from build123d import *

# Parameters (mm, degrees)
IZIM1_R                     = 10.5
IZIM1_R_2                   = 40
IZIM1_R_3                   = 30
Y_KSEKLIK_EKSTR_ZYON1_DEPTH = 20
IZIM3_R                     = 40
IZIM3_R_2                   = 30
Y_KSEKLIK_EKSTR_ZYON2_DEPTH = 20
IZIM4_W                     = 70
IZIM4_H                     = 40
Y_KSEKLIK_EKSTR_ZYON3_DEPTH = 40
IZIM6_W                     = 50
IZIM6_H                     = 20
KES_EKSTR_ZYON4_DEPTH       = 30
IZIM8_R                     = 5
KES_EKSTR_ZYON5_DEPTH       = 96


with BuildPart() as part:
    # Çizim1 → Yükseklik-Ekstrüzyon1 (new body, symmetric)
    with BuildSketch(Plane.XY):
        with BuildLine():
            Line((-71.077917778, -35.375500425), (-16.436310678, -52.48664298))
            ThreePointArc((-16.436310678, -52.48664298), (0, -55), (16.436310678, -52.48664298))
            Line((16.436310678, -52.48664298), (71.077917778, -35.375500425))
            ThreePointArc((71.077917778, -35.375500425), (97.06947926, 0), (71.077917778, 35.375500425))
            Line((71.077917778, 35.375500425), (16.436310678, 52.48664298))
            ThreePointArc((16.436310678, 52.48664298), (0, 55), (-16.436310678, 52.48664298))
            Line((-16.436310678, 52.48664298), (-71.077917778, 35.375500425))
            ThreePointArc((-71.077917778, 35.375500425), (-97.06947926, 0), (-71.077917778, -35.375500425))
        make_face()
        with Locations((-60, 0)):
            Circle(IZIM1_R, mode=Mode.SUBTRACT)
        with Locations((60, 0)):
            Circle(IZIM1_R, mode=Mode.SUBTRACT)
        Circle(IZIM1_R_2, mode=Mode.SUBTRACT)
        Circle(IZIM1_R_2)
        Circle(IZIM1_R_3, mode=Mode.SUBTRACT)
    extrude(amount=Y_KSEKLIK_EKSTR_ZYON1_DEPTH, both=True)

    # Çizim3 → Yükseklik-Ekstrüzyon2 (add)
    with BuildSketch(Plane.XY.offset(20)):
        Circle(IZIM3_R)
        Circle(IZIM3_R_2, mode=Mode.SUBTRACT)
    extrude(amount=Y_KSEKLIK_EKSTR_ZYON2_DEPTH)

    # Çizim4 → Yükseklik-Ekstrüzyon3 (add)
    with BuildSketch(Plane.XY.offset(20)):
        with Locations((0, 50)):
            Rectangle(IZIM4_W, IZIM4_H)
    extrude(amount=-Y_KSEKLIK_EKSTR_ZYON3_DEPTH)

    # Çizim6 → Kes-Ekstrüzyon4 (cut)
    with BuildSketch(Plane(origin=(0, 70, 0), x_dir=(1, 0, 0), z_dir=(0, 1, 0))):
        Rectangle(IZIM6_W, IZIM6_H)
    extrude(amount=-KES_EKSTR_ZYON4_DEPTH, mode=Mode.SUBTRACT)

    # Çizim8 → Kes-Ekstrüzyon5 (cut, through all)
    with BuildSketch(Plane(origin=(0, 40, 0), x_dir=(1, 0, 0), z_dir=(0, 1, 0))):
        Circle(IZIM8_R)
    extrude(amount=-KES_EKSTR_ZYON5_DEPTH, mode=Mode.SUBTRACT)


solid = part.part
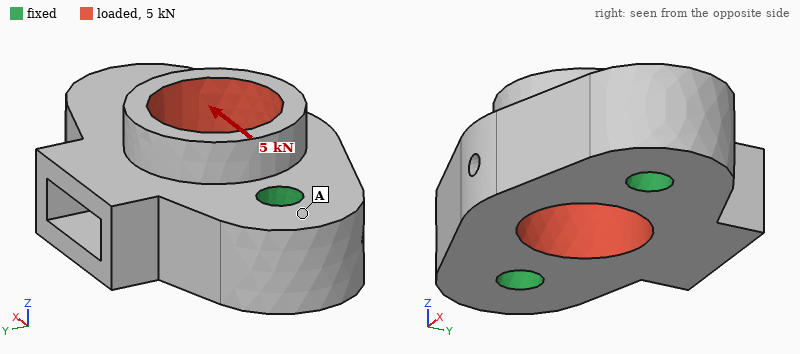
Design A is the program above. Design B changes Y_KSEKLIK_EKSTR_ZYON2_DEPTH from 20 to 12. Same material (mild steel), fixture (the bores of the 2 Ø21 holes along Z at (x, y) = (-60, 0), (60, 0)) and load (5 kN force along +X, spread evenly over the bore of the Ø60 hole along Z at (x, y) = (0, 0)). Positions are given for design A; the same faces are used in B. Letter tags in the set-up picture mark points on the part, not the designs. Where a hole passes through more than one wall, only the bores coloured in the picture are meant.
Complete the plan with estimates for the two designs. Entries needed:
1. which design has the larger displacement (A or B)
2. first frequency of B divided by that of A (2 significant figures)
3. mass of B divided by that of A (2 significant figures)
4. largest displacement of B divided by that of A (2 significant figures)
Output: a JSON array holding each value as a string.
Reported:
["A", "1.0", "0.97", "0.71"]
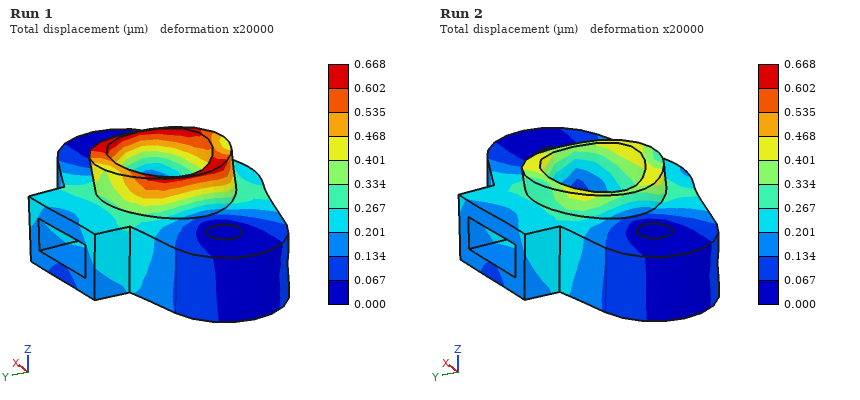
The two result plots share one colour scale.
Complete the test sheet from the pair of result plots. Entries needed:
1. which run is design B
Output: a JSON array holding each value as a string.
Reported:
["Run 2"]
